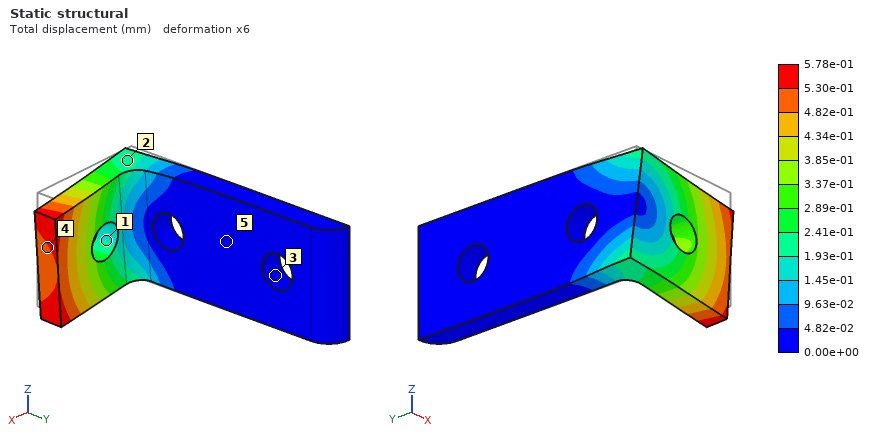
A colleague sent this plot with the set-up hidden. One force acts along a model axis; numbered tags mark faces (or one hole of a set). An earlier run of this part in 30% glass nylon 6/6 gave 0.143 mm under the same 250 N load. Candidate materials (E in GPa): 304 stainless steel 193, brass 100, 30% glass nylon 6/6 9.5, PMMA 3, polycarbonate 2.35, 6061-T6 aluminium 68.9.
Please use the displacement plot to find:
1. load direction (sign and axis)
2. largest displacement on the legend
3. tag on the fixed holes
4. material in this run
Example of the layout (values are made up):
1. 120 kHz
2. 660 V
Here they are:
1. -Z
2. 5.78e-01 mm
3. 3
4. polycarbonate
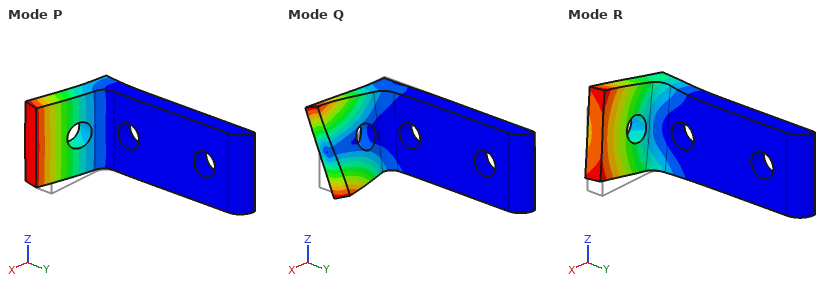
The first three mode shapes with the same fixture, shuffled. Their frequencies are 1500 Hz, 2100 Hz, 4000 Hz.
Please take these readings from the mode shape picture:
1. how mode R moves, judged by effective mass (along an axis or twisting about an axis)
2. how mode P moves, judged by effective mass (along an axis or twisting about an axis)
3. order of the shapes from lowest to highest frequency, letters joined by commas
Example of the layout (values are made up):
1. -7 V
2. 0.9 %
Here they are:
1. along Z
2. along Y
3. P, R, Q
